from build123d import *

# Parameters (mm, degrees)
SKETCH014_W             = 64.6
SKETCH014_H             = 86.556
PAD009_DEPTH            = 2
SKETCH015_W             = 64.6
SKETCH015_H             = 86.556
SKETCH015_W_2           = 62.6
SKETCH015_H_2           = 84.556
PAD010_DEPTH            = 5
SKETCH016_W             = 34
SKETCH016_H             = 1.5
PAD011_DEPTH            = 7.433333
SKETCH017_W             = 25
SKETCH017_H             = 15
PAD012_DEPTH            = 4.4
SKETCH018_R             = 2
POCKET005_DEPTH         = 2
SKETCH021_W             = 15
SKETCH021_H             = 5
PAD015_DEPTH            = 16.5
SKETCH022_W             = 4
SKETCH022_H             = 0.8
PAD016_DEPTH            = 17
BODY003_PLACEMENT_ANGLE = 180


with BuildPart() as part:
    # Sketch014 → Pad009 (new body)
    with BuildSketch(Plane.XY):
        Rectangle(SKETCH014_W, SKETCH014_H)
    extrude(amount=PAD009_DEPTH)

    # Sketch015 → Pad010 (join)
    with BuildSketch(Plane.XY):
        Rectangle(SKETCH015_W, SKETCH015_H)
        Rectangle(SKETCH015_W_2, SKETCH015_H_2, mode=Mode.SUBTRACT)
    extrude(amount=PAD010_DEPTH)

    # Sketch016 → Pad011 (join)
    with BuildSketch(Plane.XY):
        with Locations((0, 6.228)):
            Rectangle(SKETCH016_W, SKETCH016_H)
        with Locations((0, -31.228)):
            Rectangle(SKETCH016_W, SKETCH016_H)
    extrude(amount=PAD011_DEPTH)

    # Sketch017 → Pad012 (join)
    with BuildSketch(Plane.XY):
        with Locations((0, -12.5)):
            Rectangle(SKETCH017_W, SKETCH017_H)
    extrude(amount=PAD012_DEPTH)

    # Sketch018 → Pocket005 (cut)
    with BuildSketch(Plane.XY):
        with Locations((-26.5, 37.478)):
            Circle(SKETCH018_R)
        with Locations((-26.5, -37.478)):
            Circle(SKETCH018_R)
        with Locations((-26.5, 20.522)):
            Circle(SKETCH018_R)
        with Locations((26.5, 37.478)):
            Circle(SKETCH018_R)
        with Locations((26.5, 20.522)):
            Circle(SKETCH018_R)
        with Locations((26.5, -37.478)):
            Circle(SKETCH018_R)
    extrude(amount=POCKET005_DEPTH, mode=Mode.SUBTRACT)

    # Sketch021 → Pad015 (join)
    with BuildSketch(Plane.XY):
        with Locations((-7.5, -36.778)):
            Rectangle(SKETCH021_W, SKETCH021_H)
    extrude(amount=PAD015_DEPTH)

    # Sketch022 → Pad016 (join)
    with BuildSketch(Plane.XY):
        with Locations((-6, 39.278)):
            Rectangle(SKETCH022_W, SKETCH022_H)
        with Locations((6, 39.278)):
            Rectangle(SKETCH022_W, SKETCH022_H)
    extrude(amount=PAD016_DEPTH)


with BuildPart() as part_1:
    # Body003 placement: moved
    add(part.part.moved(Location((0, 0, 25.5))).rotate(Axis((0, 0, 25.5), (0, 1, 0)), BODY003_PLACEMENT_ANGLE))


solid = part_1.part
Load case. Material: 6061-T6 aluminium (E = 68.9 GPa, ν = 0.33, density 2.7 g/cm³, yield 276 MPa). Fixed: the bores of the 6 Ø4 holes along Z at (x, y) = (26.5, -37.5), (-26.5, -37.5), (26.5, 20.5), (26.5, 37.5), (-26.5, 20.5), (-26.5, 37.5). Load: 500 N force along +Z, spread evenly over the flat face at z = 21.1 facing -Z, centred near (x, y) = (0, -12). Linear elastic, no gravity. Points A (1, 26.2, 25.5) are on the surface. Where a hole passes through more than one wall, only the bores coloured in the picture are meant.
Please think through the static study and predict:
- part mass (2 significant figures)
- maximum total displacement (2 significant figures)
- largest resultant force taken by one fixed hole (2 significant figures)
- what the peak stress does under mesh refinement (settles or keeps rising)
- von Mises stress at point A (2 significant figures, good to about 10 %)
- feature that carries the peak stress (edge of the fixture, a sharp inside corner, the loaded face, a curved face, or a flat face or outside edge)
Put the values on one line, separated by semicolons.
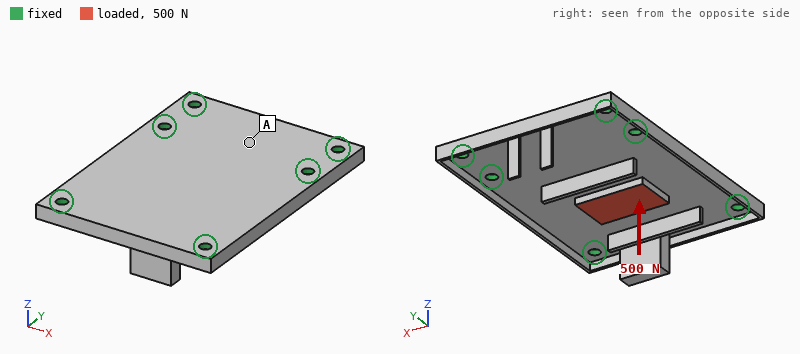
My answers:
39 g; 0.15 mm; 180 N; keeps rising; 14 MPa; edge of the fixture
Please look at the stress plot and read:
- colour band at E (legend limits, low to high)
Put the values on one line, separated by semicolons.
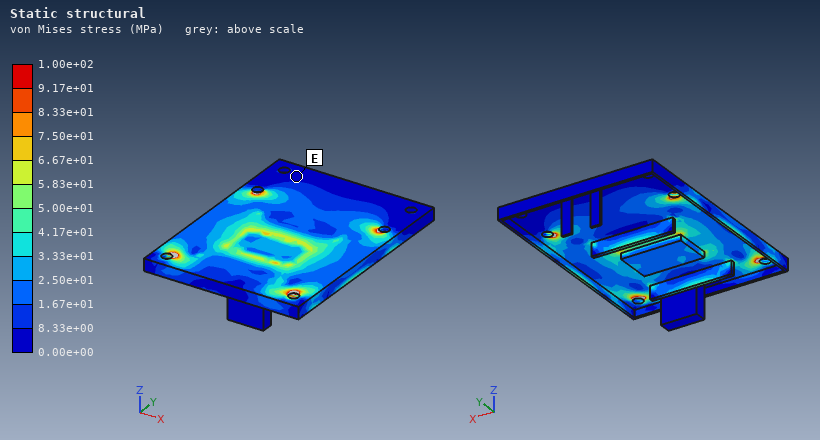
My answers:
0.00e+00 to 8.33e+00 MPa
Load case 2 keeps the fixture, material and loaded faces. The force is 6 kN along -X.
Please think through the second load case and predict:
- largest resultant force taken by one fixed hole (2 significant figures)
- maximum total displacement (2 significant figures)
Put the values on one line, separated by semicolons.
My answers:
2.0 kN; 0.19 mm
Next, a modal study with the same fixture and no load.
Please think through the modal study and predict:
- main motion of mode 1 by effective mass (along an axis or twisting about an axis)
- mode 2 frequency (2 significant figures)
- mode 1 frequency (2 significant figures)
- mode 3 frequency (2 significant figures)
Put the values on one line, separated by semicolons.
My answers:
along Z; 2800 Hz; 2700 Hz; 2900 Hz
